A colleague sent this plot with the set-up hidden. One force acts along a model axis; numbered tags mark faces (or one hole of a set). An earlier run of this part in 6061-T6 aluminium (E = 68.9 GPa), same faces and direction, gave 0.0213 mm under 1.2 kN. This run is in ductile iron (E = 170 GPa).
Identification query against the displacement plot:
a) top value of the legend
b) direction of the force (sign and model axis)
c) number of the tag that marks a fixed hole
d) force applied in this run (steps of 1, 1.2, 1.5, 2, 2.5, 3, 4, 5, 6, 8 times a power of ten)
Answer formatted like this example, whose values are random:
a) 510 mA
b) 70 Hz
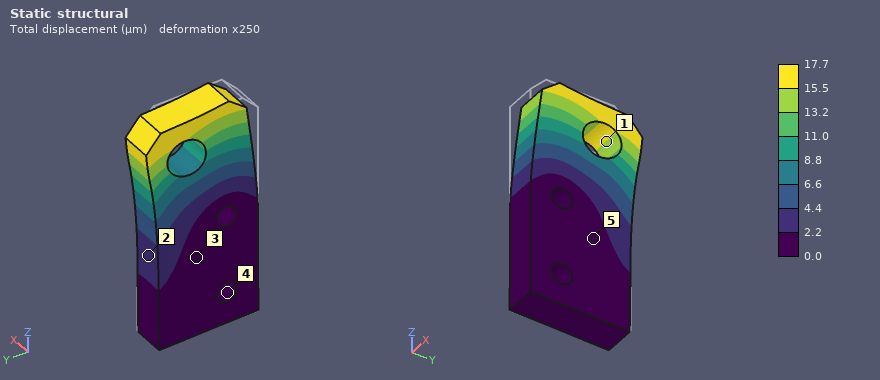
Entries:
a) 17.7 µm
b) +Y
c) 4
d) 2.5 kN
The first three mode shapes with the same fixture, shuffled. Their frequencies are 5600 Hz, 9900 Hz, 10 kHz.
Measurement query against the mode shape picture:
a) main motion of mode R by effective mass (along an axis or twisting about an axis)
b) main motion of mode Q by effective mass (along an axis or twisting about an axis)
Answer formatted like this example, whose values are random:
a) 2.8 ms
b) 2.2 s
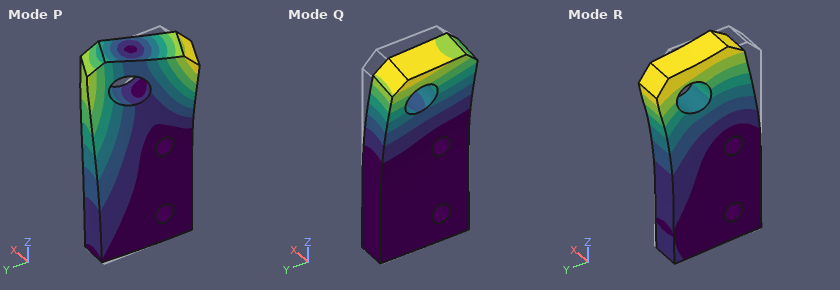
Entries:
a) along Y
b) along X
